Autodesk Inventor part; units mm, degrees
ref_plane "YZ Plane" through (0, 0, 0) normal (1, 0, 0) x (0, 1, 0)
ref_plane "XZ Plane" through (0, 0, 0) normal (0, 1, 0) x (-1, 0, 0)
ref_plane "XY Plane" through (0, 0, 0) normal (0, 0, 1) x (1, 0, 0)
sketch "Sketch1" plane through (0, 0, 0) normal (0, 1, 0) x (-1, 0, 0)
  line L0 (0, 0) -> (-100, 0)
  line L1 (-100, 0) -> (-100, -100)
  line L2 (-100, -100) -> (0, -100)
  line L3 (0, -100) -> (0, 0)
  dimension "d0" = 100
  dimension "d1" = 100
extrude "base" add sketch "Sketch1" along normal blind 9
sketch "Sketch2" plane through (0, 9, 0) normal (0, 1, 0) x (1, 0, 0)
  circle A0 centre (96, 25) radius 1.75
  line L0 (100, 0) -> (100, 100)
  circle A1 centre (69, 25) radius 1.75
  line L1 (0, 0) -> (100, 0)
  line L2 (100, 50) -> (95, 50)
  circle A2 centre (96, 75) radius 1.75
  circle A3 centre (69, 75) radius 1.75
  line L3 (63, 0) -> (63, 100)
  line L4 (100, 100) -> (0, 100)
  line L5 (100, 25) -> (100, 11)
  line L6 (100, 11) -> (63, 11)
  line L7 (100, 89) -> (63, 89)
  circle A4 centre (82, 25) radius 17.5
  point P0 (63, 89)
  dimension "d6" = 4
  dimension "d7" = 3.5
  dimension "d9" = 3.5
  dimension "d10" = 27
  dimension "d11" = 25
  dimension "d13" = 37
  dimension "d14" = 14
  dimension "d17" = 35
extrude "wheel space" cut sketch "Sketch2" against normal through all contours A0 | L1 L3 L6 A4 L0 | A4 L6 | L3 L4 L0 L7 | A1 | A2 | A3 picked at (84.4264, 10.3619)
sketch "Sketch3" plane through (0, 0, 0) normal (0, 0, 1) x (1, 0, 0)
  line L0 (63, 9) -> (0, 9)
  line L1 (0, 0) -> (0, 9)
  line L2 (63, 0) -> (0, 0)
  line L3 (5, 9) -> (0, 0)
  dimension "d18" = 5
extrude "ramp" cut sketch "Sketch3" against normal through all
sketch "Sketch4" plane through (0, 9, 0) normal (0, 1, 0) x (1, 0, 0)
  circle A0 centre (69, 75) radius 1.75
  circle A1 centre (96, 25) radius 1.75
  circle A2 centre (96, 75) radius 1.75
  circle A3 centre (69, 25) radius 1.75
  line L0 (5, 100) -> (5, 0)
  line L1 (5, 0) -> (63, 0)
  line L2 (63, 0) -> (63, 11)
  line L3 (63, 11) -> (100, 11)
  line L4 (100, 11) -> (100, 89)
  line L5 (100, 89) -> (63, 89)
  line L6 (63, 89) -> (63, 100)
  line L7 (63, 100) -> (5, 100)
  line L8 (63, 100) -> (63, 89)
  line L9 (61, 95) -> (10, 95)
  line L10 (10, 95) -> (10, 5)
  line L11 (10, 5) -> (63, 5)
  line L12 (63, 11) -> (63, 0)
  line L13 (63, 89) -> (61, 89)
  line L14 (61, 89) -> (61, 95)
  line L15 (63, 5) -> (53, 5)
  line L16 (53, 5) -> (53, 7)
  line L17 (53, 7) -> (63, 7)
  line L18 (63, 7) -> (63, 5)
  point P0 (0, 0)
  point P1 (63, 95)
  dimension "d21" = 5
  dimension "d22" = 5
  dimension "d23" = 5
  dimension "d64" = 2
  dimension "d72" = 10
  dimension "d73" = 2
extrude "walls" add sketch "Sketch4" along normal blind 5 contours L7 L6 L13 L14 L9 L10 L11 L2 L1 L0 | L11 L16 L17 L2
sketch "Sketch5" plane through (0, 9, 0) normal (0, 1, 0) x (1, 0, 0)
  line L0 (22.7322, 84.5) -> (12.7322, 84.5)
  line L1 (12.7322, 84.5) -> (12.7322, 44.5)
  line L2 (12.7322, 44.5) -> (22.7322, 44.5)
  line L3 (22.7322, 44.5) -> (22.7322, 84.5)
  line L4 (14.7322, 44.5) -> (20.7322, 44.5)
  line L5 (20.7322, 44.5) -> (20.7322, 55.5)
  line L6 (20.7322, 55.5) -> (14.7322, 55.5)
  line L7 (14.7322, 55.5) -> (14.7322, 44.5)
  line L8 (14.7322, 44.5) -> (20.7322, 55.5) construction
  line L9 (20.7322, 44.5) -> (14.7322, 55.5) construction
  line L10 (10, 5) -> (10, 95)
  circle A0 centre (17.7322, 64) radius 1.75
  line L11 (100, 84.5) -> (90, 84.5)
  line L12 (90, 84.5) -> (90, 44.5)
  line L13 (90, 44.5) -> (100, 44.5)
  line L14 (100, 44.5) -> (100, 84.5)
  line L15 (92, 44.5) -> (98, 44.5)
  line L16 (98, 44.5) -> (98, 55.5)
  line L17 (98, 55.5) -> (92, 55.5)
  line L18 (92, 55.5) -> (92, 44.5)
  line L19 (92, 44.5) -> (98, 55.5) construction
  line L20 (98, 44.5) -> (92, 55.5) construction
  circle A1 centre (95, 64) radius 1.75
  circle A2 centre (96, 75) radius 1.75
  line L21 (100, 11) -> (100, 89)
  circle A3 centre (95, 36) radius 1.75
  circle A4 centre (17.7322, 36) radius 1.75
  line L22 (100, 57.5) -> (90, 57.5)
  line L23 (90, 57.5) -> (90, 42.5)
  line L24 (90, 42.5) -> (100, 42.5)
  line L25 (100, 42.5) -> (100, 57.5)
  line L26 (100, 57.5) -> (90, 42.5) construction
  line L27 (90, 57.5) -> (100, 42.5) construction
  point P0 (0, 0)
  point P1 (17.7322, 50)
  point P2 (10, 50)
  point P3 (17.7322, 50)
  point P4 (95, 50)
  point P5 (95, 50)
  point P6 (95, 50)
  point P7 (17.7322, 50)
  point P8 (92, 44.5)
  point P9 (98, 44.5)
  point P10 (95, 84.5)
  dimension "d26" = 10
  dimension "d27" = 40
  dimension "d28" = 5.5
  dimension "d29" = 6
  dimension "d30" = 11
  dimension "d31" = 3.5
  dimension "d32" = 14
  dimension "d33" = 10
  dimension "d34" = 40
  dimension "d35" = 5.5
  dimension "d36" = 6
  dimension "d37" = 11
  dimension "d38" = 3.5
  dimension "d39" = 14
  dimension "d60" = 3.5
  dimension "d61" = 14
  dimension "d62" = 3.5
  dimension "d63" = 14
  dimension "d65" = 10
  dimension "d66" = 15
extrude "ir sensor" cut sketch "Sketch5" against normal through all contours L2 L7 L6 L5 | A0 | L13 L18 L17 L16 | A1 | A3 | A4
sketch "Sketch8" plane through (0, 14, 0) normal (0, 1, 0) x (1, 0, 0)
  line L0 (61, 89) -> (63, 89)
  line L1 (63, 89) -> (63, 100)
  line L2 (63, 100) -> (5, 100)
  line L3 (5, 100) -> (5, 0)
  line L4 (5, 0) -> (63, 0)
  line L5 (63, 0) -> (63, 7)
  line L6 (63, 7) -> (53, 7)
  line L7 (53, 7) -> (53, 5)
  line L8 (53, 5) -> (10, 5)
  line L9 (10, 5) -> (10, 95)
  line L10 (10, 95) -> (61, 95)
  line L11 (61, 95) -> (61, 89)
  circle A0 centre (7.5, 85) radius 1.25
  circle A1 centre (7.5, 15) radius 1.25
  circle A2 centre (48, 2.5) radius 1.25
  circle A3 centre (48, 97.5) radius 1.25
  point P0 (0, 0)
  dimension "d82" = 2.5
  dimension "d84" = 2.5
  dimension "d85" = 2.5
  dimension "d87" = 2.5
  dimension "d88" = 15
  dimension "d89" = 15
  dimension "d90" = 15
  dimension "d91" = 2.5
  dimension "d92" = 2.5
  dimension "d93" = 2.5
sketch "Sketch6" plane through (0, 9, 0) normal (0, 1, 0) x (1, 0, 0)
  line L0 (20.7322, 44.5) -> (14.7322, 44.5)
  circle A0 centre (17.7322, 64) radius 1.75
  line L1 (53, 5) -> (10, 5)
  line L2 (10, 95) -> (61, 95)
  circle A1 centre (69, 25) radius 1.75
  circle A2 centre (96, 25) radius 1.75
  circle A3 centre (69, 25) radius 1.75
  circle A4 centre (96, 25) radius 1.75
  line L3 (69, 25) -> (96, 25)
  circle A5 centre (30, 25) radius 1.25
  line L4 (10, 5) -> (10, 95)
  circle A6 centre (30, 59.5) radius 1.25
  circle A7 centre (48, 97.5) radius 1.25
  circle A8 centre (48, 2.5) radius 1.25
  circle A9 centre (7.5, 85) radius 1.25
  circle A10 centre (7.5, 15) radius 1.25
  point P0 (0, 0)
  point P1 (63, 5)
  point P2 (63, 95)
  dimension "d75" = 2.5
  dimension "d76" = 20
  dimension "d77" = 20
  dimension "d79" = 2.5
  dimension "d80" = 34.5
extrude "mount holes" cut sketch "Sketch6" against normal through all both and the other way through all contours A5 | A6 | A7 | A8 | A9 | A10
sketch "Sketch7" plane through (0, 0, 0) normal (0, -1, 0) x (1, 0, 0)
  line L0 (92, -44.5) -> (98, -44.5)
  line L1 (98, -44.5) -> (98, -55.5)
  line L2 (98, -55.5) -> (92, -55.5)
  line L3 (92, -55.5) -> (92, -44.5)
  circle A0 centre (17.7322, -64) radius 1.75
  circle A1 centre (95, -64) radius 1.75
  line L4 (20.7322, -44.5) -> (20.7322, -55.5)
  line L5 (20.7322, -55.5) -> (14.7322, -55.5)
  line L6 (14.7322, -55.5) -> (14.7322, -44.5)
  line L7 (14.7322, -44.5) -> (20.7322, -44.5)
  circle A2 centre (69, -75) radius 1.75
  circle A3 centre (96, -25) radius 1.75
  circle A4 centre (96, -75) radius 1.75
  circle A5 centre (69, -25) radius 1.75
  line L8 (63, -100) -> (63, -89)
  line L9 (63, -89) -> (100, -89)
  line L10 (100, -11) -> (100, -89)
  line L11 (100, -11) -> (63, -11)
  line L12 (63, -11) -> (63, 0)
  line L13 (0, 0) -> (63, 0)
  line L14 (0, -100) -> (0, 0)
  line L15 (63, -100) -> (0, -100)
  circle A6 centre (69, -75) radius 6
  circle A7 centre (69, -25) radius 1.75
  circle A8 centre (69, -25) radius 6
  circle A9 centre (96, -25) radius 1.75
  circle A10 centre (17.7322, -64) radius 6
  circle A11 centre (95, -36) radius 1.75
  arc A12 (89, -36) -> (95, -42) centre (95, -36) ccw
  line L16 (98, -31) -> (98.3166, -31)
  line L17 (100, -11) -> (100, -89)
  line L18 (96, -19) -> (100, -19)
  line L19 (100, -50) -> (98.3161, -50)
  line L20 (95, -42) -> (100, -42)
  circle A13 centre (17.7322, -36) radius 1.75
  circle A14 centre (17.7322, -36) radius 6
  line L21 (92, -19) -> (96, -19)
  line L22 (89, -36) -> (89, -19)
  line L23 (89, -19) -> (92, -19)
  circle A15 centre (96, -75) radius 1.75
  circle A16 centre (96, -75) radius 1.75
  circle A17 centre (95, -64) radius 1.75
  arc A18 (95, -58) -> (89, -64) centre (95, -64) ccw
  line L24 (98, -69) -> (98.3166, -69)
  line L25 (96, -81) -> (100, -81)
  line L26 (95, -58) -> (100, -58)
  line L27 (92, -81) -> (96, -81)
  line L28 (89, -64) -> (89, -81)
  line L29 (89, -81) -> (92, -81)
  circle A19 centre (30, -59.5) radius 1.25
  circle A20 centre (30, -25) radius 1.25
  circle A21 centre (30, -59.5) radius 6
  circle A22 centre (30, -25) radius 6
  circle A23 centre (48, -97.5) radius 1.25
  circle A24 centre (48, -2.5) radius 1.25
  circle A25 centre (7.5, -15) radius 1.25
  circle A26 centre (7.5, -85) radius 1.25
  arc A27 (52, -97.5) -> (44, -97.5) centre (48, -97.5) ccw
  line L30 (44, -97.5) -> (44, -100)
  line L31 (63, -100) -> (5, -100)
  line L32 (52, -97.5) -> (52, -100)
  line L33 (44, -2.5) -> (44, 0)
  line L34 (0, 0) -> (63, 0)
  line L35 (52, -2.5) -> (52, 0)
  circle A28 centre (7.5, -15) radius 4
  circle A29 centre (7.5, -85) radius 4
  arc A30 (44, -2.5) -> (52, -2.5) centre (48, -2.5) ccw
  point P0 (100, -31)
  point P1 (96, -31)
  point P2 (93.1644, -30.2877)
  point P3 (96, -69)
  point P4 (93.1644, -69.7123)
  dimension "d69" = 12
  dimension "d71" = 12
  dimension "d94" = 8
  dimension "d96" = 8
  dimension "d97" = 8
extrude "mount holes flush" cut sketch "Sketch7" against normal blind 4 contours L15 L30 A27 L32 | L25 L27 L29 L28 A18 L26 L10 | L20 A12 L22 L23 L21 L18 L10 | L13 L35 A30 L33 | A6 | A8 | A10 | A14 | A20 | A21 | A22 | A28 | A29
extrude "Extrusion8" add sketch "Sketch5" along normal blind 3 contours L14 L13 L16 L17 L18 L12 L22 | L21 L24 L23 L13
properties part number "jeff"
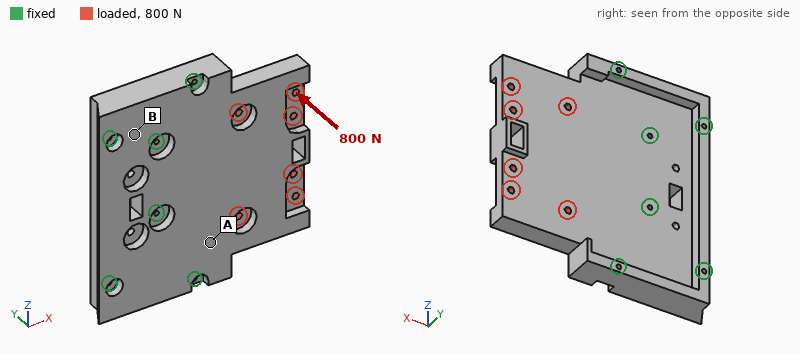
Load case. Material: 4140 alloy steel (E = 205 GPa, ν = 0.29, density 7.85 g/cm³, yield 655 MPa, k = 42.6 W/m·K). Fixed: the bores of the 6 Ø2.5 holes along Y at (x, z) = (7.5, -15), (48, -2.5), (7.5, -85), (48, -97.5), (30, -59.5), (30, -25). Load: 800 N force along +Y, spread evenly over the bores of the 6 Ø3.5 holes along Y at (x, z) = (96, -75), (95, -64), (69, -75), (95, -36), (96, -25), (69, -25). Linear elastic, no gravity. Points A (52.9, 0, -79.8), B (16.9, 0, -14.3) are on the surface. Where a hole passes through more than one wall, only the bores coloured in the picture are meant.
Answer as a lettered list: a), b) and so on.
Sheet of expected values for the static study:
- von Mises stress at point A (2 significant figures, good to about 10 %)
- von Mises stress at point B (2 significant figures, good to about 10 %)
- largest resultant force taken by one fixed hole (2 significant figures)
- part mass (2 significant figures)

a) 23 MPa
b) 5.1 MPa
c) 780 N
d) 620 g
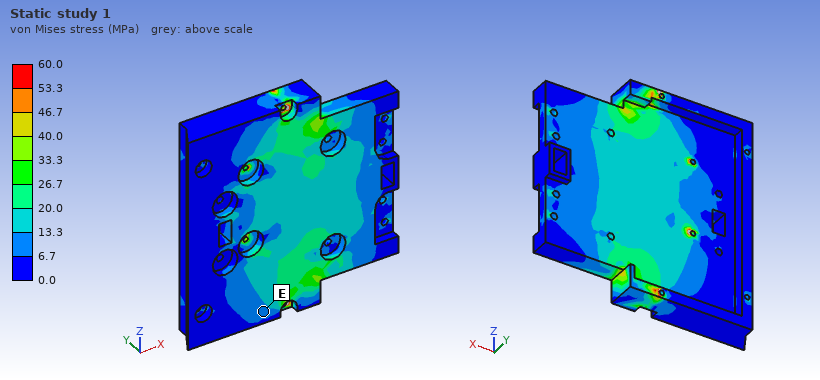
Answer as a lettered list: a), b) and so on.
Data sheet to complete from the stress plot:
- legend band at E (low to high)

a) 6.7 to 13.3 MPa
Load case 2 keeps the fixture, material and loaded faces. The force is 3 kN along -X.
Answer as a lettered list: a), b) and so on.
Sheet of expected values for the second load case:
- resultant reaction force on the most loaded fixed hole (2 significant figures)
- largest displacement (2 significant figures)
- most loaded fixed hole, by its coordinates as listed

a) 800 N
b) 8.6 µm
c) (30, -59.5)
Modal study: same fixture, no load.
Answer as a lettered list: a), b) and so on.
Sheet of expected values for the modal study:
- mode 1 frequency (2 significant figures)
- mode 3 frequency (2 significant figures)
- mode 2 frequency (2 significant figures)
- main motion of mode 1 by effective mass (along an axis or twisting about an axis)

a) 2000 Hz
b) 8200 Hz
c) 4400 Hz
d) along Y
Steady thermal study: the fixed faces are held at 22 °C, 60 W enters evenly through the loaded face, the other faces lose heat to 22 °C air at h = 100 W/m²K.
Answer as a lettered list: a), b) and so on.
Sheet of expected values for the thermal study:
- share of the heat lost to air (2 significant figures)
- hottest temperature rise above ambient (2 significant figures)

a) 68 %
b) 70 K
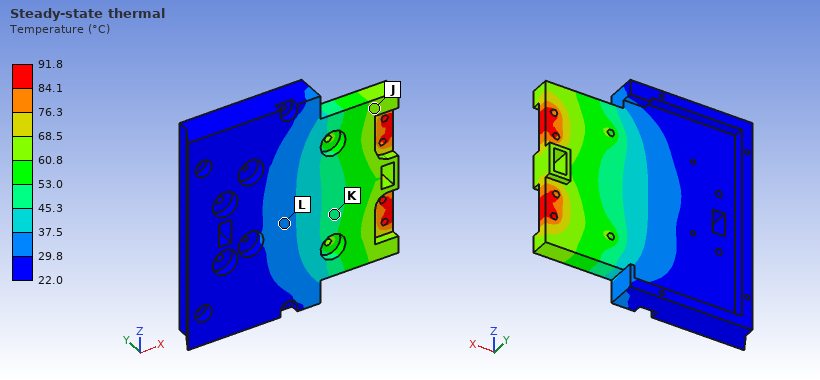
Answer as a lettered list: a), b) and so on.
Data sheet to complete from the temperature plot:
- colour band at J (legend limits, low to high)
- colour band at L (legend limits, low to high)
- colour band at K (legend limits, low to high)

a) 60.8 to 68.5 °C
b) 29.8 to 37.5 °C
c) 45.3 to 53.0 °C
